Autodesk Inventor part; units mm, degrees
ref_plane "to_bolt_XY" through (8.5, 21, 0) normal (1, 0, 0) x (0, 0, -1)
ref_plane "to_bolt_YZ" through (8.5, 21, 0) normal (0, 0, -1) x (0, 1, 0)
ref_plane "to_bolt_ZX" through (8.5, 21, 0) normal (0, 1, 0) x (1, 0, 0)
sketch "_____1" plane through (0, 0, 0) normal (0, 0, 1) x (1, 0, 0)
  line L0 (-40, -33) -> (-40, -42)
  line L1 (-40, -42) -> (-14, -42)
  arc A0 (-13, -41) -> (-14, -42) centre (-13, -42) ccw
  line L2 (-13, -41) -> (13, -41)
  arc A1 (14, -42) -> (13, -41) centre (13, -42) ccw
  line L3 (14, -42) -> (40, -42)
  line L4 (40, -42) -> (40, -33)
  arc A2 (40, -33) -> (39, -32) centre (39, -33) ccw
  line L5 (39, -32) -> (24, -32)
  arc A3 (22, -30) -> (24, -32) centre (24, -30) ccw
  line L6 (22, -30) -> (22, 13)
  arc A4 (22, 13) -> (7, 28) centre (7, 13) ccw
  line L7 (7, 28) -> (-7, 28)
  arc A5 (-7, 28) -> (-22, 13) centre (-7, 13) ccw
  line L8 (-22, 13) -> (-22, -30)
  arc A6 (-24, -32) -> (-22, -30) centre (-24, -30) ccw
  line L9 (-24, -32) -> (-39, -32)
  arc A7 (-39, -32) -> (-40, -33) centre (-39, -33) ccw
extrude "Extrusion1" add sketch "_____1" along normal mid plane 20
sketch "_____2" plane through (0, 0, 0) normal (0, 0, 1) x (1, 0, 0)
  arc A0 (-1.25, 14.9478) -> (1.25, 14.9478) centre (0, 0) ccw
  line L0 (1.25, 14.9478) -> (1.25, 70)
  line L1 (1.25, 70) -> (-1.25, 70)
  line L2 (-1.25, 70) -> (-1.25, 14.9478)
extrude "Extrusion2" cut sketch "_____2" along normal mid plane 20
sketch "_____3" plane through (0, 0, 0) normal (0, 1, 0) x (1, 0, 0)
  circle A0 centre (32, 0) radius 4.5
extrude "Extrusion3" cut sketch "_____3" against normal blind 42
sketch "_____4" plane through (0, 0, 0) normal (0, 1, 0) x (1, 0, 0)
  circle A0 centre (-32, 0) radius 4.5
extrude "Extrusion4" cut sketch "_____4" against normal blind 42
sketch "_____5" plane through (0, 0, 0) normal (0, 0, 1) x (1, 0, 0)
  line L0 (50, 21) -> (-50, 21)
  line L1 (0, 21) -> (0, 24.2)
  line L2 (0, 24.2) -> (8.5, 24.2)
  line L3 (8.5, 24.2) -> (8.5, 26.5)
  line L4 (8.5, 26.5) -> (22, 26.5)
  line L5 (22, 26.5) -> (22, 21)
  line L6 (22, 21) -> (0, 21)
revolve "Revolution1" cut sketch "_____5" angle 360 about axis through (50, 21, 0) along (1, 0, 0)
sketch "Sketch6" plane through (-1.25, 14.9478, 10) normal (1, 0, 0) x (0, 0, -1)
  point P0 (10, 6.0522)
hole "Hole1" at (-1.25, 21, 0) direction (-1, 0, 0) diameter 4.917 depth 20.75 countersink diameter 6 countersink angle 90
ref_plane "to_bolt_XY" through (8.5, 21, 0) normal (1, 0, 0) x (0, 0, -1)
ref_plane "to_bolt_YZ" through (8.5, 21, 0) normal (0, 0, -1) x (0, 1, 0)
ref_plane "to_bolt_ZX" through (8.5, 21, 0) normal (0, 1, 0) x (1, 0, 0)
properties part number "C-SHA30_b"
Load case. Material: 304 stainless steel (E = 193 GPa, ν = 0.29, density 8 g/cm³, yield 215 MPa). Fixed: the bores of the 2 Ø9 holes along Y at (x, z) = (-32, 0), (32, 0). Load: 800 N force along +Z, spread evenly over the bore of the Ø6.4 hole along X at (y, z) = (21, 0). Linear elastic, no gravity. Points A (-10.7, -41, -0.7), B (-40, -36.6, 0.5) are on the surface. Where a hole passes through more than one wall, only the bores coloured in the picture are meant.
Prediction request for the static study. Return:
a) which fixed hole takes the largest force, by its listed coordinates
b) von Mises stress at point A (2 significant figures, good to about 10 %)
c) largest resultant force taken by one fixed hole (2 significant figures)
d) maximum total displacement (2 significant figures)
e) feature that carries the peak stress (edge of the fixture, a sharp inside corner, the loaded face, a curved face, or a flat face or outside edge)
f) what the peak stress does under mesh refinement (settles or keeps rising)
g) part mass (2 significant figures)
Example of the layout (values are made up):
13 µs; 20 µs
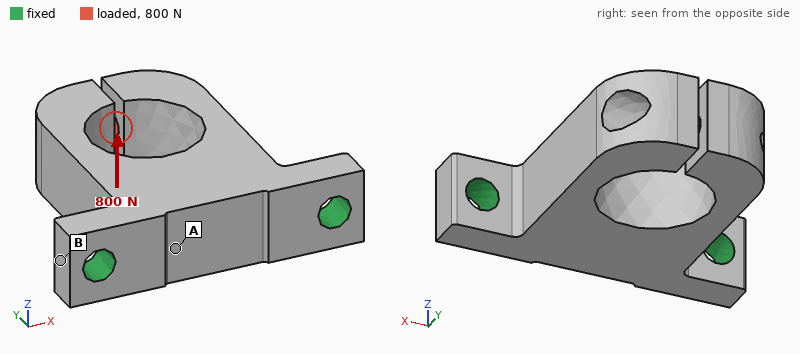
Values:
(32, 0); 16 MPa; 460 N; 96 µm; edge of the fixture; keeps rising; 390 g
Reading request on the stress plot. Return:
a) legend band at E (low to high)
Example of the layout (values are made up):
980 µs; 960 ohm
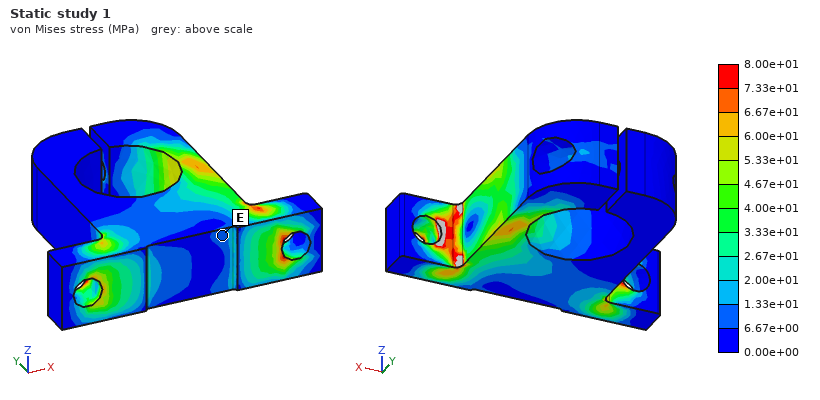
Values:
6.67e+00 to 1.33e+01 MPa
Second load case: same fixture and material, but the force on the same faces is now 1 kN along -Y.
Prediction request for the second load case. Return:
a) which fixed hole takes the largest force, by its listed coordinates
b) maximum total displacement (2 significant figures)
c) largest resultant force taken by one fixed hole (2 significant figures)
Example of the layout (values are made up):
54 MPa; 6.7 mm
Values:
(32, 0); 72 µm; 680 N
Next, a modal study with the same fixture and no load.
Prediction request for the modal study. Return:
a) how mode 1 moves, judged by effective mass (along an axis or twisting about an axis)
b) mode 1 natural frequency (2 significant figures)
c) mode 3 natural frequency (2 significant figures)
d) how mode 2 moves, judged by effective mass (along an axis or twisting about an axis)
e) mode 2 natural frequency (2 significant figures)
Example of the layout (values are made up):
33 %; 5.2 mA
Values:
along Z; 2000 Hz; 2700 Hz; along X; 2500 Hz
